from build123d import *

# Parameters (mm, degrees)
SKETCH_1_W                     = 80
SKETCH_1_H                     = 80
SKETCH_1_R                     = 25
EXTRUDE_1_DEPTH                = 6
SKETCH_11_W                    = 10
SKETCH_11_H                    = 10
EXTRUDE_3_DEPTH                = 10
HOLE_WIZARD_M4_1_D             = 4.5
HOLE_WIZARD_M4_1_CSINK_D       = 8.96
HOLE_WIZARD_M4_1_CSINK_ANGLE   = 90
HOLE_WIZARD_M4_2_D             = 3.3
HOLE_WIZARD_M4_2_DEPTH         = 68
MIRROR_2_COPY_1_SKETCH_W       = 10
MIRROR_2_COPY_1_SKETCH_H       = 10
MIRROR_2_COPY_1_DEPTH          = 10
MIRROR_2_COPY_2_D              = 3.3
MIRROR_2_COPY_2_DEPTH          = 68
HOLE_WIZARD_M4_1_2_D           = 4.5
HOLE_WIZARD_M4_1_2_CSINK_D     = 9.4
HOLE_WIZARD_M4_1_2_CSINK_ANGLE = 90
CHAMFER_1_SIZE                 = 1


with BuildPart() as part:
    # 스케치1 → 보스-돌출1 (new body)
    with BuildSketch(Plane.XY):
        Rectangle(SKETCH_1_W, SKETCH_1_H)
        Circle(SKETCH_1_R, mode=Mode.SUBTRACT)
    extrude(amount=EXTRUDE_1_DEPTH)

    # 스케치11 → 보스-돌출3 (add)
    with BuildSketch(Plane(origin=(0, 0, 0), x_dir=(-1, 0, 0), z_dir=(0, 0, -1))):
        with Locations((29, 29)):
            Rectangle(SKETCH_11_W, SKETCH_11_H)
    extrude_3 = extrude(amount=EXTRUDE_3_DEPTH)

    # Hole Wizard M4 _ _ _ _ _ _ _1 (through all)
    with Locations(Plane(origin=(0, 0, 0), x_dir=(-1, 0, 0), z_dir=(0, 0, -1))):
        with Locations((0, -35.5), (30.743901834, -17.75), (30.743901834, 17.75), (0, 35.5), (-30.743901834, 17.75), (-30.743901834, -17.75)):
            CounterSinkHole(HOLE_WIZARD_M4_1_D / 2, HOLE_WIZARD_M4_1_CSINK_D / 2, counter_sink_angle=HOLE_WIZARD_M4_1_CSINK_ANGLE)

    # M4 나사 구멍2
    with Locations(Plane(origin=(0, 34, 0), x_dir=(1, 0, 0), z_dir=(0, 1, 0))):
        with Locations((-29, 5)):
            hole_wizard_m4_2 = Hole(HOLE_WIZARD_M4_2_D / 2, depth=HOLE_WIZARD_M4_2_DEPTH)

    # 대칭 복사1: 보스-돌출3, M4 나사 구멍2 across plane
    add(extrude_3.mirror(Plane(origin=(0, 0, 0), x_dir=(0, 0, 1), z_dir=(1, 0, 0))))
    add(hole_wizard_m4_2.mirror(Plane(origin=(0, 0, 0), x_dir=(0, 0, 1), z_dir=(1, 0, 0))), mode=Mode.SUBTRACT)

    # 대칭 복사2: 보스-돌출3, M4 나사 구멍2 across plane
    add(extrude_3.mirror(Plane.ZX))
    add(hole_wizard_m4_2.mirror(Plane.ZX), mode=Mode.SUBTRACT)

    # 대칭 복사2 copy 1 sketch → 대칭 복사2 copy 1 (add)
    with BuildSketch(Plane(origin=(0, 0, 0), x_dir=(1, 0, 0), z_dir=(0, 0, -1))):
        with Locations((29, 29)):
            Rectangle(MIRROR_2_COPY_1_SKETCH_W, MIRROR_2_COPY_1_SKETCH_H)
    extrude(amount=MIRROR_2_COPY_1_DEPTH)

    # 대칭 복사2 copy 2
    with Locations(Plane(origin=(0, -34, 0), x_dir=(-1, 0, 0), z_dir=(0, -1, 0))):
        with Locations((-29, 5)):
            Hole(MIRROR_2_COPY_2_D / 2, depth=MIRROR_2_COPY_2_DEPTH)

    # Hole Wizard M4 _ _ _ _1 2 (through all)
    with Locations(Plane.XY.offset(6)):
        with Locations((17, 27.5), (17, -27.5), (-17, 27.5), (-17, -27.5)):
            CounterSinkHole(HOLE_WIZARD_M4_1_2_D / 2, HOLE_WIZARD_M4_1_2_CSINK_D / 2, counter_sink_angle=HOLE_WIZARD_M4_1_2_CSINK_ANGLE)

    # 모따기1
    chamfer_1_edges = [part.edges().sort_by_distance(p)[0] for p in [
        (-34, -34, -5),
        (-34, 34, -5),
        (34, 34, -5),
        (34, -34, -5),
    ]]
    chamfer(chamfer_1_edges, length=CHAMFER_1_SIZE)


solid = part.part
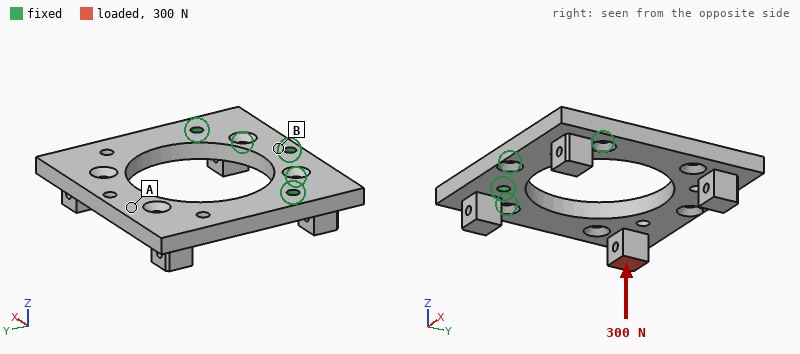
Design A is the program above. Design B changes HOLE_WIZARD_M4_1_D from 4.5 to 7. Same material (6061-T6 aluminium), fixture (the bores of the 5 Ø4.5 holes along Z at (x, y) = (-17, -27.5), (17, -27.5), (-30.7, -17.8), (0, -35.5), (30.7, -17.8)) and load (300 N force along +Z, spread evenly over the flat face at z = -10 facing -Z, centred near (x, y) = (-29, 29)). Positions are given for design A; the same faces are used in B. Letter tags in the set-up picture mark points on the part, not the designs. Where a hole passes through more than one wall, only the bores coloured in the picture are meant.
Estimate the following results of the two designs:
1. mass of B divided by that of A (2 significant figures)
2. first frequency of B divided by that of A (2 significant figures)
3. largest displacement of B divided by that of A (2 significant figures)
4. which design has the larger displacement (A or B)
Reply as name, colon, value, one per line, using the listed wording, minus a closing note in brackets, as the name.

mass of B divided by that of A: 0.98
first frequency of B divided by that of A: 1.1
largest displacement of B divided by that of A: 0.86
which design has the larger displacement: A
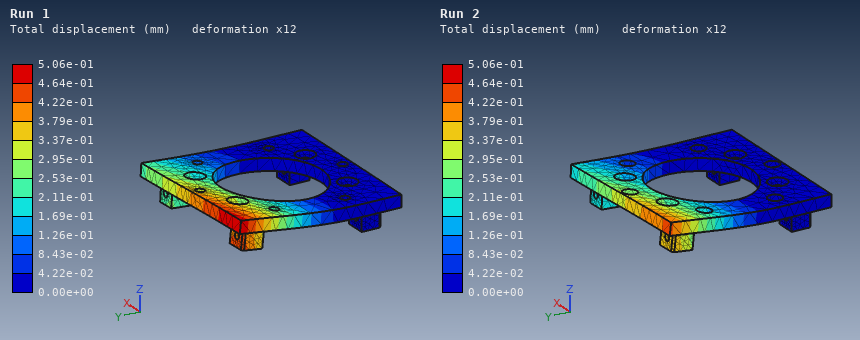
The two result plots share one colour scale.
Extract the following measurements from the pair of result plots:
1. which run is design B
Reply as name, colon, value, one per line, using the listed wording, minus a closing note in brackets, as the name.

which run is design B: Run 2
